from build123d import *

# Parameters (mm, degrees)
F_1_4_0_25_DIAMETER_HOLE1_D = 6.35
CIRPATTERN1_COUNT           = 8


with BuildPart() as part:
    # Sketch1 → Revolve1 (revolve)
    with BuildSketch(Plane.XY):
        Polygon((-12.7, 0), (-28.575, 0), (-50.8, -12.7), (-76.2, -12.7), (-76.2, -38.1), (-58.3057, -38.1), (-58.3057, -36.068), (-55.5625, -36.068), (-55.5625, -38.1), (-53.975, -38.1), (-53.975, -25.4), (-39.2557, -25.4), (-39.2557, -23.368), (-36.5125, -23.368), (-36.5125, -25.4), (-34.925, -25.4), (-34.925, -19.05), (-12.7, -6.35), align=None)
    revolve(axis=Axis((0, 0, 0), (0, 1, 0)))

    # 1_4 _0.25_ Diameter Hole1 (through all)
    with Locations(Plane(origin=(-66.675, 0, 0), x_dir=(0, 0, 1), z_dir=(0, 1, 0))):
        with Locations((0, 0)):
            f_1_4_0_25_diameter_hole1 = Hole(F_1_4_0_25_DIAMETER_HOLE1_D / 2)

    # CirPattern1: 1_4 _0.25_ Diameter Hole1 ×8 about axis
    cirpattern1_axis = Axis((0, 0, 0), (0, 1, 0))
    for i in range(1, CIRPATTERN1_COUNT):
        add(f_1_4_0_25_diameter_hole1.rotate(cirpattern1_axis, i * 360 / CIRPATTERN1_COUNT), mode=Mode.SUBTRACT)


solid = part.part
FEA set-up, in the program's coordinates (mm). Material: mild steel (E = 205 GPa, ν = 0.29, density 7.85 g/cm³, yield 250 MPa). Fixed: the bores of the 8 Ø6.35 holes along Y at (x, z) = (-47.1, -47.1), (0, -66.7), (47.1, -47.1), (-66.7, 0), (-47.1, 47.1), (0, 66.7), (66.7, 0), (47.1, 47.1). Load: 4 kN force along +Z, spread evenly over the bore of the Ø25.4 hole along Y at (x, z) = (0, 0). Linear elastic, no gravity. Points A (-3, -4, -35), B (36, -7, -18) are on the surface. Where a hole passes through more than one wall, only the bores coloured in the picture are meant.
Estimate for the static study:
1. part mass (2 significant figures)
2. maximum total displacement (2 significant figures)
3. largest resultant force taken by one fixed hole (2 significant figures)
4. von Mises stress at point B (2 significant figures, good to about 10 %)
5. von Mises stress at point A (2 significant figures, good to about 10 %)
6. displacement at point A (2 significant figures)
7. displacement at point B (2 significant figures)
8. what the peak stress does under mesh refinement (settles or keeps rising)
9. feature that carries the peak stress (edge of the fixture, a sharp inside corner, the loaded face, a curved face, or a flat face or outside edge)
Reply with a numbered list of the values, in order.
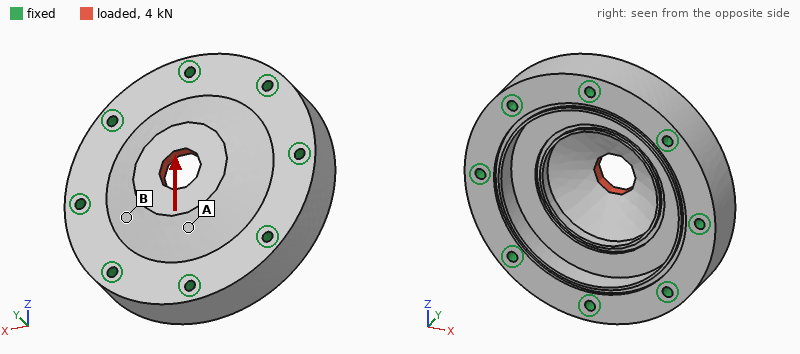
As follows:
1. 2.7 kg
2. 1.6 µm
3. 810 N
4. 1.5 MPa
5. 3.5 MPa
6. 0.67 µm
7. 0.30 µm
8. keeps rising
9. a sharp inside corner
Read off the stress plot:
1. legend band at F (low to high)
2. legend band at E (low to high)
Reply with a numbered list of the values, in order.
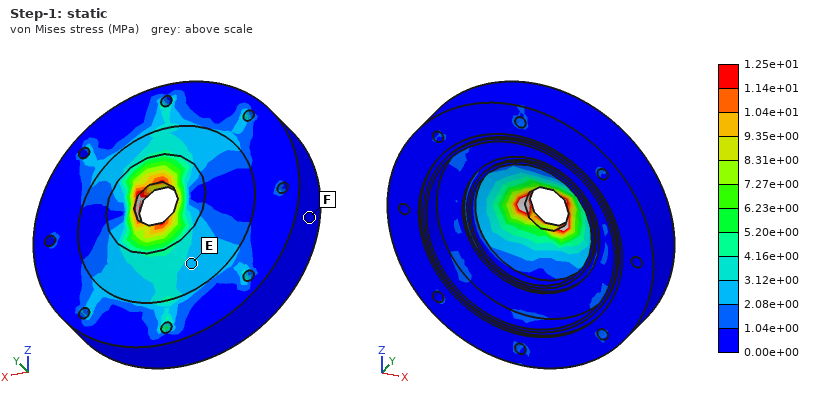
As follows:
1. 0.00e+00 to 1.04e+00 MPa
2. 2.08e+00 to 3.12e+00 MPa
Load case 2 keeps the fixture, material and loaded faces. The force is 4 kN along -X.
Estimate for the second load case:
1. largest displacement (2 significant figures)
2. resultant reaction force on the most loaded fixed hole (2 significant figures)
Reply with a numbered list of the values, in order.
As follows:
1. 1.7 µm
2. 810 N
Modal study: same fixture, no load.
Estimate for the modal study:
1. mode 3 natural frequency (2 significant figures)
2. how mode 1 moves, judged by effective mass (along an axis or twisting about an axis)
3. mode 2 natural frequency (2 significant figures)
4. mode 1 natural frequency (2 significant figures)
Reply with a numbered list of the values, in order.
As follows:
1. 14 kHz
2. along Y
3. 14 kHz
4. 11 kHz
